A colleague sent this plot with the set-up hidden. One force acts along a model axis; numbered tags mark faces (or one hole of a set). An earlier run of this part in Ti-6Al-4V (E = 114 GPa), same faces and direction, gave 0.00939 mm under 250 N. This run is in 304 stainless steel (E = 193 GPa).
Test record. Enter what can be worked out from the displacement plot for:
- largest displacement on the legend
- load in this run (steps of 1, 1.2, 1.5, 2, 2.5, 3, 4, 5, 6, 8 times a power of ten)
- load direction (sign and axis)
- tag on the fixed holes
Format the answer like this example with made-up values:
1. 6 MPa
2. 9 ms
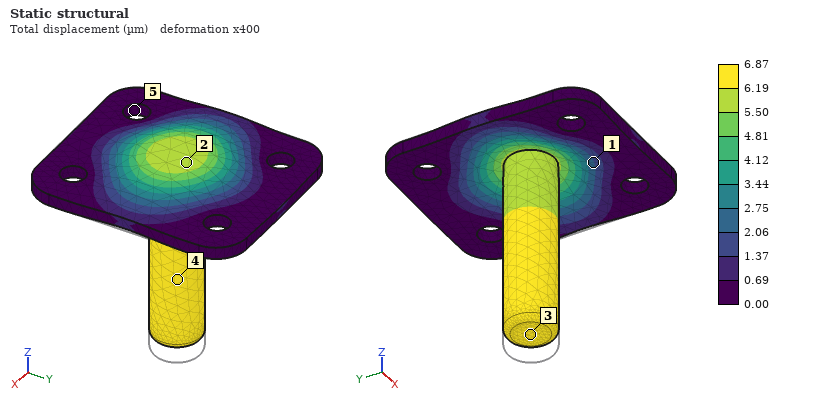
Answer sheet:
1. 6.87 µm
2. 300 N
3. +Z
4. 5
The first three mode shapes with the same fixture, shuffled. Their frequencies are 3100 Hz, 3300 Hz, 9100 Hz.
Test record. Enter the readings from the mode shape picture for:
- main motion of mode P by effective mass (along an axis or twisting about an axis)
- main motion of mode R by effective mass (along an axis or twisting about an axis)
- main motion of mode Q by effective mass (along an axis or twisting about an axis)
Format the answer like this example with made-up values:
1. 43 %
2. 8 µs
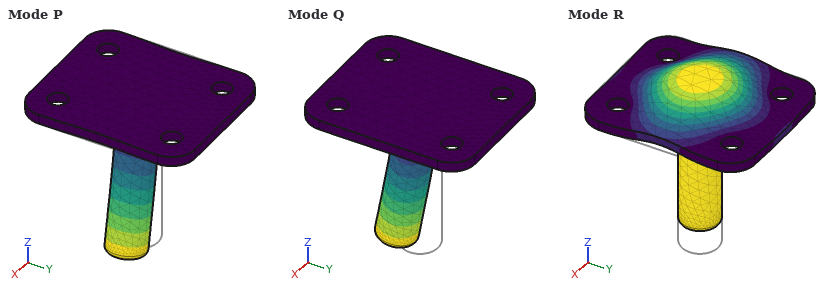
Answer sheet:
1. along X
2. along Z
3. along Y
